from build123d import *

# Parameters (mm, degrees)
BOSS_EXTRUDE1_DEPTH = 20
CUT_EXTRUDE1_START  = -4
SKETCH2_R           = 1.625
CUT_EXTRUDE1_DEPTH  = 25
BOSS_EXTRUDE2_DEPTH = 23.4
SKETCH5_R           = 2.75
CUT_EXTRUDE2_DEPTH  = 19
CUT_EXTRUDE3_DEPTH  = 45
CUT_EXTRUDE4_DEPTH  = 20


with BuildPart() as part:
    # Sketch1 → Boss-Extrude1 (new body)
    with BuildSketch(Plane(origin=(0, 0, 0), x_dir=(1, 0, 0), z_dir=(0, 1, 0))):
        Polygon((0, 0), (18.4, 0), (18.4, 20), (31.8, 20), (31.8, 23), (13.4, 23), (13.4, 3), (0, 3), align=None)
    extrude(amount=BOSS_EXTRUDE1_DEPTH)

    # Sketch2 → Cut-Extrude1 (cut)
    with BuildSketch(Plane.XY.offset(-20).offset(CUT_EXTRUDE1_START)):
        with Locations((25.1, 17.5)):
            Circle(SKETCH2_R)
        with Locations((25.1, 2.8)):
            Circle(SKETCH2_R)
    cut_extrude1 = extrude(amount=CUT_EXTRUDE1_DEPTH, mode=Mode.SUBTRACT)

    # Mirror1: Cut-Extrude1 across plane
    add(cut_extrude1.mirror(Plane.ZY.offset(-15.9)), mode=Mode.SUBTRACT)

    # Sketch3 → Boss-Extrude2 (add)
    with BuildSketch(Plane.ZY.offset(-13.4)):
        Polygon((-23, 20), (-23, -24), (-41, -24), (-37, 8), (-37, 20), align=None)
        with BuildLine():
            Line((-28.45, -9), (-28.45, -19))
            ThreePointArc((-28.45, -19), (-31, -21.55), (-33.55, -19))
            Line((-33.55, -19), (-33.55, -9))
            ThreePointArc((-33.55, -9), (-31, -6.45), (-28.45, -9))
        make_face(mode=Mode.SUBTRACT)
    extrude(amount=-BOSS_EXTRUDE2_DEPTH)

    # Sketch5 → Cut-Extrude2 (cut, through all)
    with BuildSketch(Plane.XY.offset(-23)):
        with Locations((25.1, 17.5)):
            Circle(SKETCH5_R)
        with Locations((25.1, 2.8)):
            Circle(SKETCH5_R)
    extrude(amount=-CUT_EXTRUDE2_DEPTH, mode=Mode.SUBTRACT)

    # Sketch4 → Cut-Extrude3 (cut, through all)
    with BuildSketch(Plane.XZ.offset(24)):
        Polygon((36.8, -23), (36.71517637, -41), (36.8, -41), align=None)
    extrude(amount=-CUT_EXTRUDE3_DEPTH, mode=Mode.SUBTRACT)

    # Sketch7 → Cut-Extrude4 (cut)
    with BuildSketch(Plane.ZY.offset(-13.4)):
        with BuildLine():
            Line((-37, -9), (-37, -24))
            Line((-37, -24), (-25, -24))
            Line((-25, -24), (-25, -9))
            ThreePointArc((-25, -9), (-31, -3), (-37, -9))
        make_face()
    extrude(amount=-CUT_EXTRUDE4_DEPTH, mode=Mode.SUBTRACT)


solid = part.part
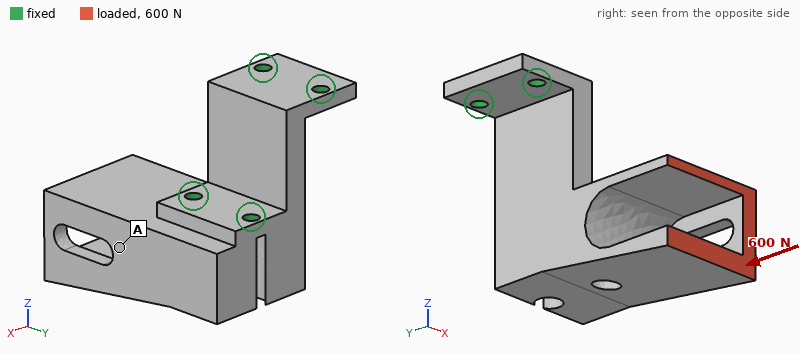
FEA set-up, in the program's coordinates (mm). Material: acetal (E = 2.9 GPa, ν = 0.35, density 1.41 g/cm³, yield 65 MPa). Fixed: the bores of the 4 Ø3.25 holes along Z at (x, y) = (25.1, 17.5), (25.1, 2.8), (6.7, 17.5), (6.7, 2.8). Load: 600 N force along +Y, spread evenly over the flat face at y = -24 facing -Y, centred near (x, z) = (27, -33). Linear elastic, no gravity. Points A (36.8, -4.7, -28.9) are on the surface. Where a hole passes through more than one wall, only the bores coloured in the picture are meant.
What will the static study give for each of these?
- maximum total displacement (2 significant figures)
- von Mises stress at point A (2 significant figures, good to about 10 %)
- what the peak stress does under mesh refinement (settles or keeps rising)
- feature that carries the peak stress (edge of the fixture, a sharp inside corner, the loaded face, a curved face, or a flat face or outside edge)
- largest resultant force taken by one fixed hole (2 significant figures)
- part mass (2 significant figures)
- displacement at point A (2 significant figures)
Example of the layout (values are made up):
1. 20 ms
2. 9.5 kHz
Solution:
1. 0.55 mm
2. 4.7 MPa
3. keeps rising
4. edge of the fixture
5. 500 N
6. 20 g
7. 0.11 mm
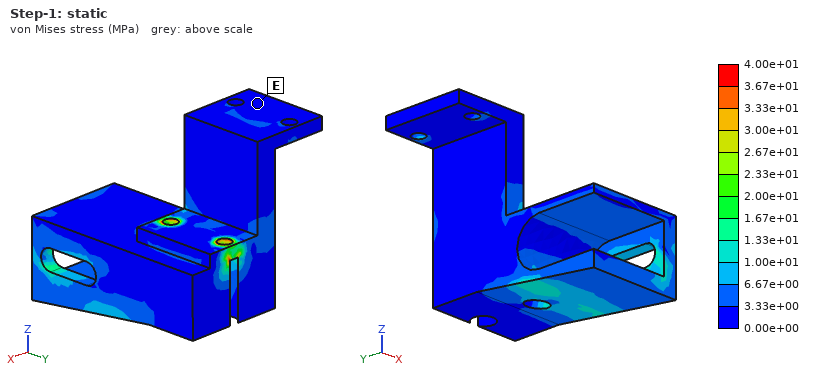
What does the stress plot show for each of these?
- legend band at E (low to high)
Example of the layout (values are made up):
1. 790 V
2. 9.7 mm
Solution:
1. 0.00e+00 to 3.33e+00 MPa
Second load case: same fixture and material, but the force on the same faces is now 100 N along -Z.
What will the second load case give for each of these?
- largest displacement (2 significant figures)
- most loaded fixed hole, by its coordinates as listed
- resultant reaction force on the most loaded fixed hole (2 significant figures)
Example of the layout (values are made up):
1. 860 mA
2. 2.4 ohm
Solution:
1. 0.81 mm
2. (25.1, 2.8)
3. 230 N
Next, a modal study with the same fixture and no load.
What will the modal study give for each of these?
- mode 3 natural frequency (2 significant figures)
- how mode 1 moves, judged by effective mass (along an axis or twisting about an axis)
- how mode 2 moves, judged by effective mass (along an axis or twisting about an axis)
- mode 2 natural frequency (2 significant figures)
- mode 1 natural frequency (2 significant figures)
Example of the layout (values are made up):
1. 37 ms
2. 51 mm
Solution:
1. 2200 Hz
2. along X
3. along Z
4. 1700 Hz
5. 1600 Hz
